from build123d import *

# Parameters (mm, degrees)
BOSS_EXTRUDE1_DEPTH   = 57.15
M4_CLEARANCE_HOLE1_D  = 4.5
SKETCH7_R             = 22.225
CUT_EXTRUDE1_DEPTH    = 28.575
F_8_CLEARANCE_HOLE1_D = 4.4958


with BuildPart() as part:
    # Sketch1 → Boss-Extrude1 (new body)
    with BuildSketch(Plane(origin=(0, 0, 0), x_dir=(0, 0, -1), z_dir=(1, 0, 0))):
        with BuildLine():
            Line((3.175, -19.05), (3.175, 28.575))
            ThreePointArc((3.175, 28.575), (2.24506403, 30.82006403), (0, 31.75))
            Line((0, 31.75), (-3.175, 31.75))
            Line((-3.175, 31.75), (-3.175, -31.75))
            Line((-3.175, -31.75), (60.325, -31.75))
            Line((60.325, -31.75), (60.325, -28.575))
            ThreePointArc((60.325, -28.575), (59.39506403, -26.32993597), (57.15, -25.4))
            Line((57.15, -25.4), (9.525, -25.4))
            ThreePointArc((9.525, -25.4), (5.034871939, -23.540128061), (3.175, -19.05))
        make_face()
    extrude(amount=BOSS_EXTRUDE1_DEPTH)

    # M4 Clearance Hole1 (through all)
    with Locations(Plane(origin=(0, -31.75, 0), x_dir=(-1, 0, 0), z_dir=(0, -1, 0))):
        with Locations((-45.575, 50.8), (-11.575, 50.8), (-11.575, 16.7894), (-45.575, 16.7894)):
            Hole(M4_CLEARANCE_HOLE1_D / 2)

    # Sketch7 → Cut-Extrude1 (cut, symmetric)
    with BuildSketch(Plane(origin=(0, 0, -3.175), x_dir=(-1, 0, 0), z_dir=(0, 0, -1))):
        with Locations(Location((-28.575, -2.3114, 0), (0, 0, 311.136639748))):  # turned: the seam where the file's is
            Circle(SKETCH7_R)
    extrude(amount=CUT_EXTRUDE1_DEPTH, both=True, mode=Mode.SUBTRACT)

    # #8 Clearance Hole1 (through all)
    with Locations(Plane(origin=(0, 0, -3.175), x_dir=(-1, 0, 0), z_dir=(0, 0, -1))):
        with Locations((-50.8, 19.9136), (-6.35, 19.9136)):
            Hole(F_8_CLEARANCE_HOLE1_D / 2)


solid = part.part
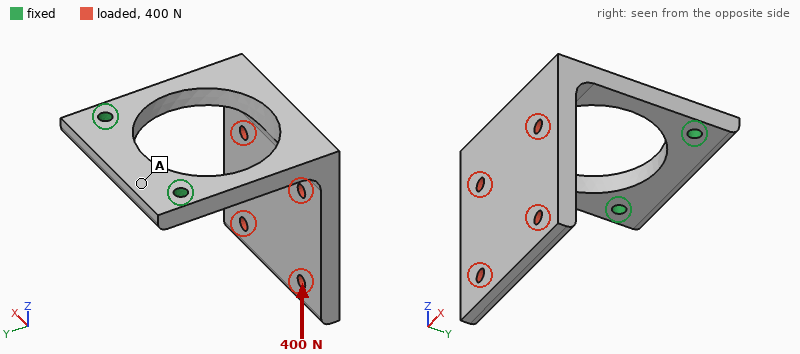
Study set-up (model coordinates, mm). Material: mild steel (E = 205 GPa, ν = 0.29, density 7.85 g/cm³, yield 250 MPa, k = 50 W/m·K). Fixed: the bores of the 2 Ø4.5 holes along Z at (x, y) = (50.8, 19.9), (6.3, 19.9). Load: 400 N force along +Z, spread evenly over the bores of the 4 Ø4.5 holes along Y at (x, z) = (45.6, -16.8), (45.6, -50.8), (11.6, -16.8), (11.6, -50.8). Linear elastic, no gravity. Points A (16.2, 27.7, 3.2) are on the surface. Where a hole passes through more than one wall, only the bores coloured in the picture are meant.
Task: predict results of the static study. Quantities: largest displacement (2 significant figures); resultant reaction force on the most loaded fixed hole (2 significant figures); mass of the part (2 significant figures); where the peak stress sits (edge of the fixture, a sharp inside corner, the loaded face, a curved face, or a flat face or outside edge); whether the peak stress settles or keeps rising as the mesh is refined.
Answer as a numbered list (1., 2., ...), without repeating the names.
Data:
1. 0.42 mm
2. 200 N
3. 260 g
4. edge of the fixture
5. keeps rising
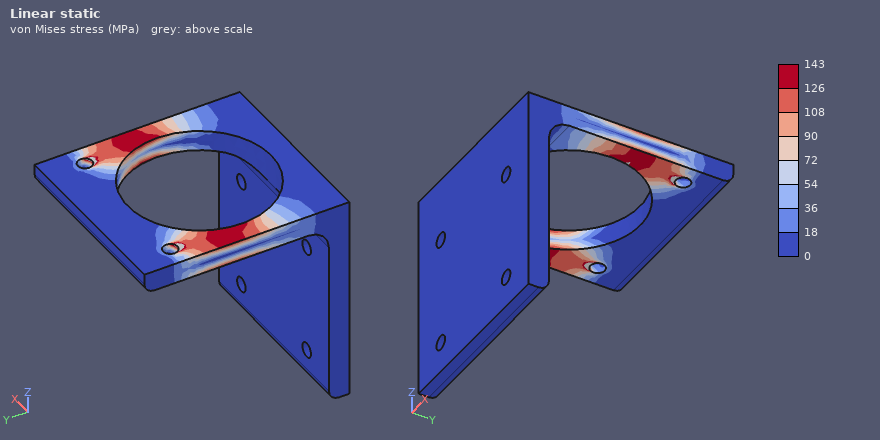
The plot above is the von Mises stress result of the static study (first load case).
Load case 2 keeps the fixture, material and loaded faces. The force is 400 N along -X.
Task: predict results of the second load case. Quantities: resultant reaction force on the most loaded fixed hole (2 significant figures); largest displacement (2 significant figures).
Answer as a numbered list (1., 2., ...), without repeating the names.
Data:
1. 460 N
2. 0.14 mm
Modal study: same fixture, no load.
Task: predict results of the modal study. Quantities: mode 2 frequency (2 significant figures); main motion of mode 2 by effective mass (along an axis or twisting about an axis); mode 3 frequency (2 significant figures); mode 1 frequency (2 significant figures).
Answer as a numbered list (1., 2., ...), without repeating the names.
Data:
1. 800 Hz
2. along X
3. 1400 Hz
4. 350 Hz
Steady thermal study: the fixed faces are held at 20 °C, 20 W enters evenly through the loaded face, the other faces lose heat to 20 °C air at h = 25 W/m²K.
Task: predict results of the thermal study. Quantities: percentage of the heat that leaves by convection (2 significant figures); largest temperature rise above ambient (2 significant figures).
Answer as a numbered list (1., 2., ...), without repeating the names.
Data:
1. 71 %
2. 69 K
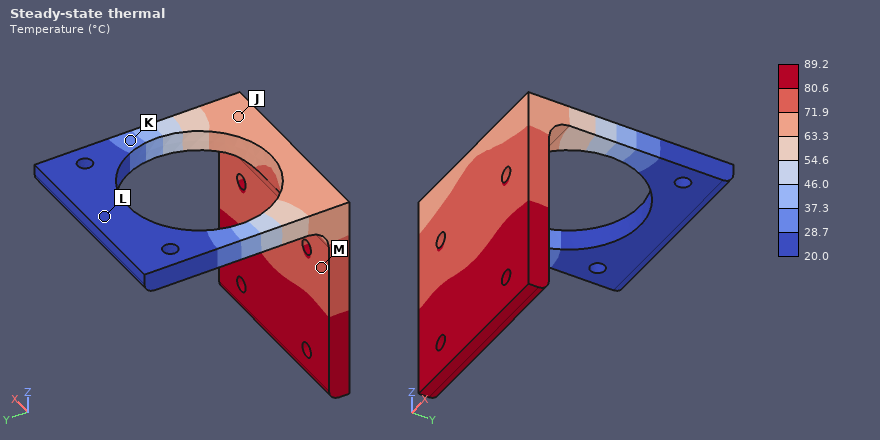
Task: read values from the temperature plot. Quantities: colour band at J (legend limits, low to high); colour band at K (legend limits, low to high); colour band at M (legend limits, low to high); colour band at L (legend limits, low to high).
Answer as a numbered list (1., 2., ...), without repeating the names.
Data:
1. 63.3 to 71.9 °C
2. 28.7 to 37.3 °C
3. 71.9 to 80.6 °C
4. 20.0 to 28.7 °C
